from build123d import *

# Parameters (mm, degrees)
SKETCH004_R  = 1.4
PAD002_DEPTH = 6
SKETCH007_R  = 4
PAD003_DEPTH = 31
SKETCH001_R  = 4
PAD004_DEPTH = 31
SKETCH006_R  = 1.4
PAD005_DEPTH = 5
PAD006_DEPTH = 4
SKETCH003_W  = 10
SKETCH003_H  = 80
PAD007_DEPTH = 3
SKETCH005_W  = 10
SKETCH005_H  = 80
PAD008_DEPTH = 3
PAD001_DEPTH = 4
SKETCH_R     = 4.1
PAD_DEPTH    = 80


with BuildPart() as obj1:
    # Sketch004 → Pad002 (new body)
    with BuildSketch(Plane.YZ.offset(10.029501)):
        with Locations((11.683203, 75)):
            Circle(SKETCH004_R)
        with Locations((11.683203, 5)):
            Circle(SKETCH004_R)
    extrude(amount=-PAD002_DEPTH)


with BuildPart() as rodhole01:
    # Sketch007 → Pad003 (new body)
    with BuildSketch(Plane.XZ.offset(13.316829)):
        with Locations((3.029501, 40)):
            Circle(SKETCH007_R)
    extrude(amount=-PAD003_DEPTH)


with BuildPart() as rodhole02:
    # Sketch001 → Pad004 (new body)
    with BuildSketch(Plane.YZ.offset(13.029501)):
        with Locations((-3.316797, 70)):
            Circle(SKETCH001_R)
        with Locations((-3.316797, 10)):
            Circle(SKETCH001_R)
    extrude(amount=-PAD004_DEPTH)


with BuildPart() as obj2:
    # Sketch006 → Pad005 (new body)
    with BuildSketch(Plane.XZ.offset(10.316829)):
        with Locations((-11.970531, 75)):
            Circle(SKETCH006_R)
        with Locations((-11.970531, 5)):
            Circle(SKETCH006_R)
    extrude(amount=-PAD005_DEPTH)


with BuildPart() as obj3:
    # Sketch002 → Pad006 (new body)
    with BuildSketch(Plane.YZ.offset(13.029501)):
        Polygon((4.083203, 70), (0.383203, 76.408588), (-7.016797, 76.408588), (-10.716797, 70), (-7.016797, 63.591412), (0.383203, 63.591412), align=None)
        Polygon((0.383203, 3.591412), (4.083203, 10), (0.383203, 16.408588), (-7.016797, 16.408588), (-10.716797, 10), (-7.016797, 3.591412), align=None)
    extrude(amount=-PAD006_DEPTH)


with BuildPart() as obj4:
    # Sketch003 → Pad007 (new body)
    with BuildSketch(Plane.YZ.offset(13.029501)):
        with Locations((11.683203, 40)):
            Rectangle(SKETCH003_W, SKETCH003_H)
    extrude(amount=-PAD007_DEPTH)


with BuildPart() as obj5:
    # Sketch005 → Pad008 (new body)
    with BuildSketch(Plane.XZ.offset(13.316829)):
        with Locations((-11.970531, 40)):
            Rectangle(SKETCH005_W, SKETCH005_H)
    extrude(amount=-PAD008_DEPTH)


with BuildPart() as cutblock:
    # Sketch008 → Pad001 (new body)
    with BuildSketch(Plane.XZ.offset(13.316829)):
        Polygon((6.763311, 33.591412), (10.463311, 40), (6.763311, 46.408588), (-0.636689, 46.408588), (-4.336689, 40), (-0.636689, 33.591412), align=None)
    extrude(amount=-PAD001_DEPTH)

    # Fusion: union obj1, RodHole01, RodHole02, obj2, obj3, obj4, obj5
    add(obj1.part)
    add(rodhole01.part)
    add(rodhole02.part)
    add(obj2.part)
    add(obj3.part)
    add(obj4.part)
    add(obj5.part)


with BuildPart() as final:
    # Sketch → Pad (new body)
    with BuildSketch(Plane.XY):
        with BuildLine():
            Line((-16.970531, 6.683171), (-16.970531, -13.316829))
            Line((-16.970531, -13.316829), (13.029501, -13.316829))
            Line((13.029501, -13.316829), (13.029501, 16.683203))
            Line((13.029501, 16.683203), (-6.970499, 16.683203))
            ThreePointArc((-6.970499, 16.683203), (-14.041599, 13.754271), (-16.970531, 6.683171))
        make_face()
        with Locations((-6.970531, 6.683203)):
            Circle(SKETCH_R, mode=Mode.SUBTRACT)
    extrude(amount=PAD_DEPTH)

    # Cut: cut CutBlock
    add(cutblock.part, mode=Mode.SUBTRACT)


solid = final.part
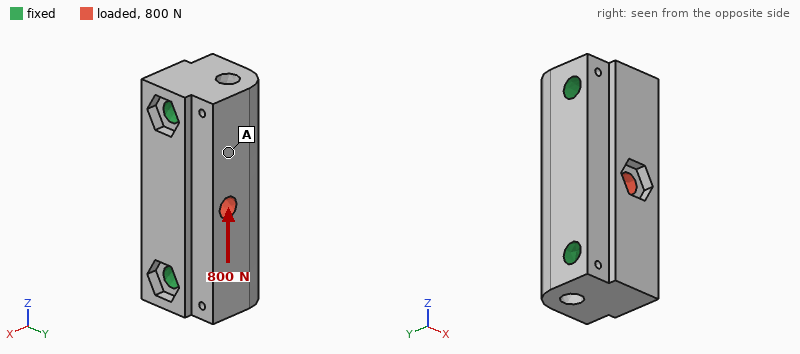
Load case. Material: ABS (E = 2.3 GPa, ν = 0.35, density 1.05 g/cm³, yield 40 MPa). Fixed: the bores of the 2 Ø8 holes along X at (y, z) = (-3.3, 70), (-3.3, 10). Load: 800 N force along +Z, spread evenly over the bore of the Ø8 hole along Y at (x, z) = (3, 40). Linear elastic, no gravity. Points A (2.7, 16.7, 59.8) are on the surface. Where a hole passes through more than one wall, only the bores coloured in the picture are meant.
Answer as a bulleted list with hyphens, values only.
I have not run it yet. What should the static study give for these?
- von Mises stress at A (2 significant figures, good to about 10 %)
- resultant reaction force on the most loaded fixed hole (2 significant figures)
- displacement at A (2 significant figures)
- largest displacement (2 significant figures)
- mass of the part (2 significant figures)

- 0.36 MPa
- 410 N
- 8.2 µm
- 15 µm
- 58 g
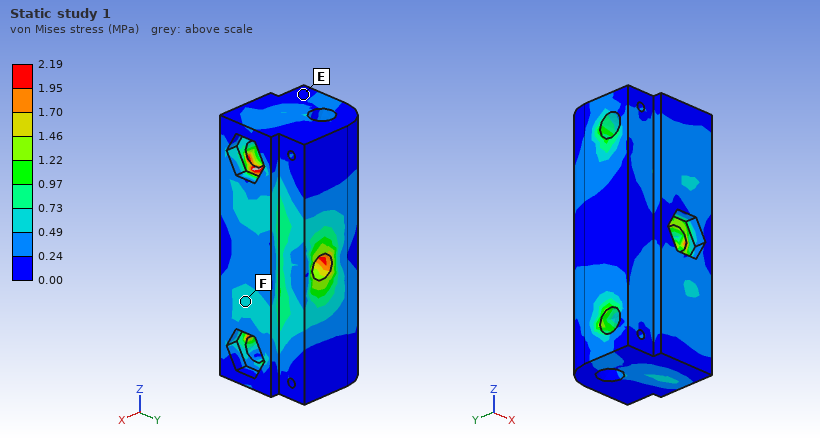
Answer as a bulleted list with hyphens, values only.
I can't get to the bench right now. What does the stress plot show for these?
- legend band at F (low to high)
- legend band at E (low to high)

- 0.49 to 0.73 MPa
- 0.00 to 0.24 MPa
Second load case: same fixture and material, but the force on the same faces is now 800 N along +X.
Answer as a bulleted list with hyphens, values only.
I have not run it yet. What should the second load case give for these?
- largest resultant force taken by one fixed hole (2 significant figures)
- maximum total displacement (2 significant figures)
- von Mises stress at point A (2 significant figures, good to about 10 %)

- 400 N
- 55 µm
- 0.89 MPa
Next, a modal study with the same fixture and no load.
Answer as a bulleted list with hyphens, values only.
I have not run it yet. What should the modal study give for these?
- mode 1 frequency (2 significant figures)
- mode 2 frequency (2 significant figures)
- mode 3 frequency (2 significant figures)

- 5000 Hz
- 5200 Hz
- 6600 Hz
